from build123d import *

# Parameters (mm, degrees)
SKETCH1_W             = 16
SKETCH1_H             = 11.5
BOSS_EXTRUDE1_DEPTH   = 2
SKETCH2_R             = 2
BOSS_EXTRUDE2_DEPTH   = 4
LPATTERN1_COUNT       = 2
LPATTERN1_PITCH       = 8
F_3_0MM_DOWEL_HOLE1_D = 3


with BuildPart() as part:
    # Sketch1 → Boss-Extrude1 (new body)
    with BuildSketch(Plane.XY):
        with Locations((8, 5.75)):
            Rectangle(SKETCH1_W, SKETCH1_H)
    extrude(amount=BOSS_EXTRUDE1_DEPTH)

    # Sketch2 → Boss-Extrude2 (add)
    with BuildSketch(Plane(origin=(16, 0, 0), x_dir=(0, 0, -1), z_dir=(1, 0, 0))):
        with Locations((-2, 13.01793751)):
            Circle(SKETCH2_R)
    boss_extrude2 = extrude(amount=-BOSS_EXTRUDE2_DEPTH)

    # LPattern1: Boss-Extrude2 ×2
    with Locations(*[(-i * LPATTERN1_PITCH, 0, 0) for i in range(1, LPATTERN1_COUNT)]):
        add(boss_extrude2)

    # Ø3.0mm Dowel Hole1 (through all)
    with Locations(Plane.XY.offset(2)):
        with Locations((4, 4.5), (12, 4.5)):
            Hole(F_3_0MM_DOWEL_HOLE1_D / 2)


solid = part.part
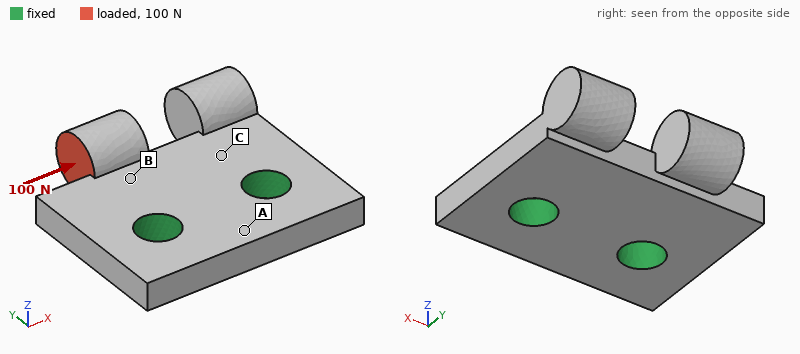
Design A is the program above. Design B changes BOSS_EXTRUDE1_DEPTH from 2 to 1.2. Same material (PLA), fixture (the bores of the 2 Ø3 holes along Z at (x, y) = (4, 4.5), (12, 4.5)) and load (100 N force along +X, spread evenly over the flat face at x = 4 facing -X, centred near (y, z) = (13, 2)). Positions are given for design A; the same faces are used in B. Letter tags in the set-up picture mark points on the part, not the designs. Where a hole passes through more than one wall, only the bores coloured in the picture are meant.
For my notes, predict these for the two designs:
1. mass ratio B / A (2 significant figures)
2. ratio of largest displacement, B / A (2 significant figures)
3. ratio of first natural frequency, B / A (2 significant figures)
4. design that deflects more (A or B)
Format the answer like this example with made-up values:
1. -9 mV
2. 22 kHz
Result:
1. 0.70
2. 3.4
3. 0.48
4. B
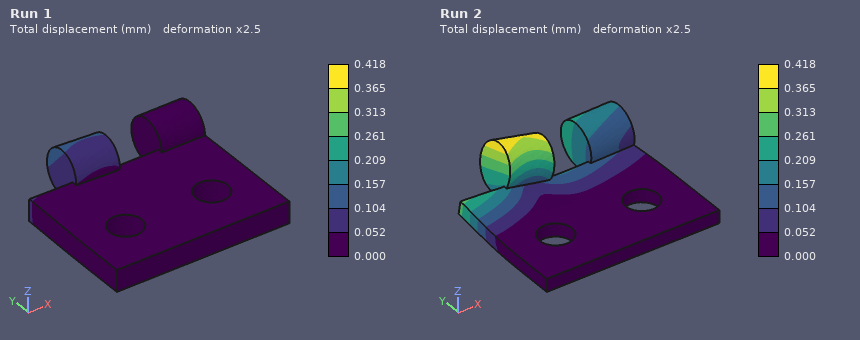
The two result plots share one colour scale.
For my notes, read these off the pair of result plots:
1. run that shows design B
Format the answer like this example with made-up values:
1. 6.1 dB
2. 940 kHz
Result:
1. Run 2
